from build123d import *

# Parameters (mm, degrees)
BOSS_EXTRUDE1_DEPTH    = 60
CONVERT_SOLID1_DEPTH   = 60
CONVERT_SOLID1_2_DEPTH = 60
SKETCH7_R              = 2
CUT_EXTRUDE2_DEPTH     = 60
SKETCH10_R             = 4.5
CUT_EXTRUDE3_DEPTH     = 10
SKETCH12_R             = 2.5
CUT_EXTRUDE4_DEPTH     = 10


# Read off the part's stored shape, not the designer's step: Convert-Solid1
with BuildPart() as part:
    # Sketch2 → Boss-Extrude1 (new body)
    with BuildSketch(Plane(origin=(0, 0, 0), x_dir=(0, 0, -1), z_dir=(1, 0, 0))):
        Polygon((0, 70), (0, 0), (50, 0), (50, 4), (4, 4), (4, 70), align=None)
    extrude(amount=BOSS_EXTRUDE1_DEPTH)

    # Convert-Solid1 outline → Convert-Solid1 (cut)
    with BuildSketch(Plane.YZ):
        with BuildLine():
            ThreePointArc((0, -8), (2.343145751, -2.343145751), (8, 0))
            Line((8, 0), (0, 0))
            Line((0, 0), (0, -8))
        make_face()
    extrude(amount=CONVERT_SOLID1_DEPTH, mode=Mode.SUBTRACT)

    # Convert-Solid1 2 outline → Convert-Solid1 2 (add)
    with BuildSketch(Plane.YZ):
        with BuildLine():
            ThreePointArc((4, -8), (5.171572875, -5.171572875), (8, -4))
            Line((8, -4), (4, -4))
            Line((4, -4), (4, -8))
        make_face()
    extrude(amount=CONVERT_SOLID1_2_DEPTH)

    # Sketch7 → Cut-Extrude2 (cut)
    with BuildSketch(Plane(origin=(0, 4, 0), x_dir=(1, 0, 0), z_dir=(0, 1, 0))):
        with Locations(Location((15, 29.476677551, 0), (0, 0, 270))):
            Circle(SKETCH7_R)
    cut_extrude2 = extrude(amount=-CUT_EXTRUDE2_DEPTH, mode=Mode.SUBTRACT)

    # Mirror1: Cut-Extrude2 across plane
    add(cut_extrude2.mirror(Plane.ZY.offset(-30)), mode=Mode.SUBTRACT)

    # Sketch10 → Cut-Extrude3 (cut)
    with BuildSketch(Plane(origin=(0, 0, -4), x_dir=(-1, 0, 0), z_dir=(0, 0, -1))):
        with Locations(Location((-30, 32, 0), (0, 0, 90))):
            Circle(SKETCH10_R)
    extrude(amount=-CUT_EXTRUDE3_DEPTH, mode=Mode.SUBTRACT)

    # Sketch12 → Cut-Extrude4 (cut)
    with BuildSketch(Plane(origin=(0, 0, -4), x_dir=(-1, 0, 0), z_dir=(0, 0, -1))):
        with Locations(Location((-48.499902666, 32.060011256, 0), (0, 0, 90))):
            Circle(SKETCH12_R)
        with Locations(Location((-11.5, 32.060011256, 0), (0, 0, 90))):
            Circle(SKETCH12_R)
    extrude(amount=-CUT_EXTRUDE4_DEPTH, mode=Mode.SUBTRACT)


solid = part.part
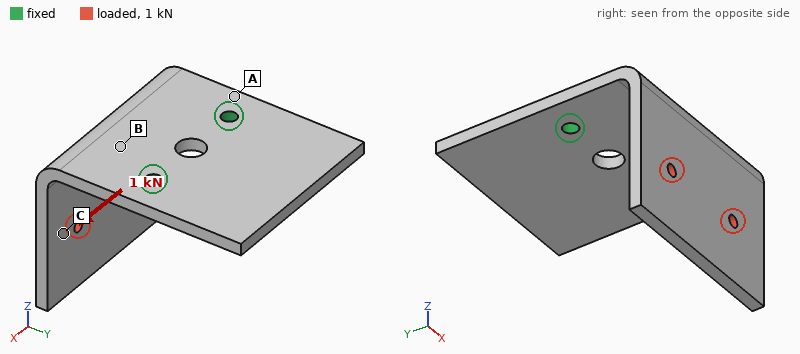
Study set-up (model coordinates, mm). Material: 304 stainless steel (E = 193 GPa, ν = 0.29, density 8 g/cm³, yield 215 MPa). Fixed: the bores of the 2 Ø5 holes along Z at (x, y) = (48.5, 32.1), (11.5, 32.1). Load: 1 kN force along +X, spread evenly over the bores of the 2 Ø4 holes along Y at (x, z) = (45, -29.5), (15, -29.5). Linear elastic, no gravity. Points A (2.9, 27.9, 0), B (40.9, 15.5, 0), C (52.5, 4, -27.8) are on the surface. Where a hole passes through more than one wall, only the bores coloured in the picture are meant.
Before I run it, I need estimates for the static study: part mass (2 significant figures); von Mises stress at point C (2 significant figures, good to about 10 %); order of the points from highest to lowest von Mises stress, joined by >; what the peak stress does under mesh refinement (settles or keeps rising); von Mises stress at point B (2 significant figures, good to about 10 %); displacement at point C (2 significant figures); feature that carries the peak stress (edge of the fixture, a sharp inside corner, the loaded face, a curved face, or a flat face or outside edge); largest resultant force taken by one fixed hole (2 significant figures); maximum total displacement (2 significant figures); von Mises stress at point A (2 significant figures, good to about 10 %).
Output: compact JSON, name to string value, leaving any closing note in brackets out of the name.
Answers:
{"part mass": "210 g", "von Mises stress at point C": "22 MPa", "order of the points from highest to lowest von Mises stress, joined by >": "A > B > C", "what the peak stress does under mesh refinement": "keeps rising", "von Mises stress at point B": "72 MPa", "displacement at point C": "0.13 mm", "feature that carries the peak stress": "edge of the fixture", "largest resultant force taken by one fixed hole": "1.1 kN", "maximum total displacement": "0.22 mm", "von Mises stress at point A": "100 MPa"}
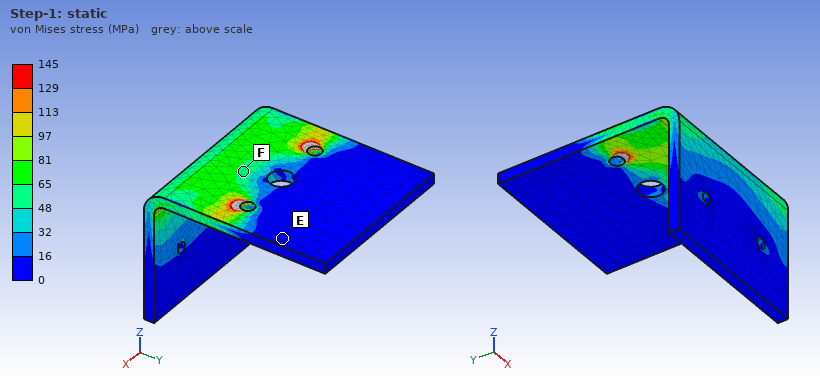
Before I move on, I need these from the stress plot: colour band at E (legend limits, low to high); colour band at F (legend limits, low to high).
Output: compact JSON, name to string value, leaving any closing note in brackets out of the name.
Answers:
{"colour band at E": "0 to 16 MPa", "colour band at F": "48 to 65 MPa"}
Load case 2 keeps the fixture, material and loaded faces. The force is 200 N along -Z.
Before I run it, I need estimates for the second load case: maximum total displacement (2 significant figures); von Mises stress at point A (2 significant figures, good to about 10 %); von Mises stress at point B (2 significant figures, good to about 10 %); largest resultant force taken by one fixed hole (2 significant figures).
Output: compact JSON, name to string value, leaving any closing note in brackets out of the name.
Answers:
{"maximum total displacement": "80 µm", "von Mises stress at point A": "27 MPa", "von Mises stress at point B": "15 MPa", "largest resultant force taken by one fixed hole": "100 N"}
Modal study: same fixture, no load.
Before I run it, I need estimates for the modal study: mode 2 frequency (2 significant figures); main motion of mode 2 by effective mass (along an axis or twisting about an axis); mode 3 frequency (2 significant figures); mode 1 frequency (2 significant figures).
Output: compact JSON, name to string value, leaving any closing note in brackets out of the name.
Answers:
{"mode 2 frequency": "1300 Hz", "main motion of mode 2 by effective mass": "along X", "mode 3 frequency": "2000 Hz", "mode 1 frequency": "690 Hz"}
